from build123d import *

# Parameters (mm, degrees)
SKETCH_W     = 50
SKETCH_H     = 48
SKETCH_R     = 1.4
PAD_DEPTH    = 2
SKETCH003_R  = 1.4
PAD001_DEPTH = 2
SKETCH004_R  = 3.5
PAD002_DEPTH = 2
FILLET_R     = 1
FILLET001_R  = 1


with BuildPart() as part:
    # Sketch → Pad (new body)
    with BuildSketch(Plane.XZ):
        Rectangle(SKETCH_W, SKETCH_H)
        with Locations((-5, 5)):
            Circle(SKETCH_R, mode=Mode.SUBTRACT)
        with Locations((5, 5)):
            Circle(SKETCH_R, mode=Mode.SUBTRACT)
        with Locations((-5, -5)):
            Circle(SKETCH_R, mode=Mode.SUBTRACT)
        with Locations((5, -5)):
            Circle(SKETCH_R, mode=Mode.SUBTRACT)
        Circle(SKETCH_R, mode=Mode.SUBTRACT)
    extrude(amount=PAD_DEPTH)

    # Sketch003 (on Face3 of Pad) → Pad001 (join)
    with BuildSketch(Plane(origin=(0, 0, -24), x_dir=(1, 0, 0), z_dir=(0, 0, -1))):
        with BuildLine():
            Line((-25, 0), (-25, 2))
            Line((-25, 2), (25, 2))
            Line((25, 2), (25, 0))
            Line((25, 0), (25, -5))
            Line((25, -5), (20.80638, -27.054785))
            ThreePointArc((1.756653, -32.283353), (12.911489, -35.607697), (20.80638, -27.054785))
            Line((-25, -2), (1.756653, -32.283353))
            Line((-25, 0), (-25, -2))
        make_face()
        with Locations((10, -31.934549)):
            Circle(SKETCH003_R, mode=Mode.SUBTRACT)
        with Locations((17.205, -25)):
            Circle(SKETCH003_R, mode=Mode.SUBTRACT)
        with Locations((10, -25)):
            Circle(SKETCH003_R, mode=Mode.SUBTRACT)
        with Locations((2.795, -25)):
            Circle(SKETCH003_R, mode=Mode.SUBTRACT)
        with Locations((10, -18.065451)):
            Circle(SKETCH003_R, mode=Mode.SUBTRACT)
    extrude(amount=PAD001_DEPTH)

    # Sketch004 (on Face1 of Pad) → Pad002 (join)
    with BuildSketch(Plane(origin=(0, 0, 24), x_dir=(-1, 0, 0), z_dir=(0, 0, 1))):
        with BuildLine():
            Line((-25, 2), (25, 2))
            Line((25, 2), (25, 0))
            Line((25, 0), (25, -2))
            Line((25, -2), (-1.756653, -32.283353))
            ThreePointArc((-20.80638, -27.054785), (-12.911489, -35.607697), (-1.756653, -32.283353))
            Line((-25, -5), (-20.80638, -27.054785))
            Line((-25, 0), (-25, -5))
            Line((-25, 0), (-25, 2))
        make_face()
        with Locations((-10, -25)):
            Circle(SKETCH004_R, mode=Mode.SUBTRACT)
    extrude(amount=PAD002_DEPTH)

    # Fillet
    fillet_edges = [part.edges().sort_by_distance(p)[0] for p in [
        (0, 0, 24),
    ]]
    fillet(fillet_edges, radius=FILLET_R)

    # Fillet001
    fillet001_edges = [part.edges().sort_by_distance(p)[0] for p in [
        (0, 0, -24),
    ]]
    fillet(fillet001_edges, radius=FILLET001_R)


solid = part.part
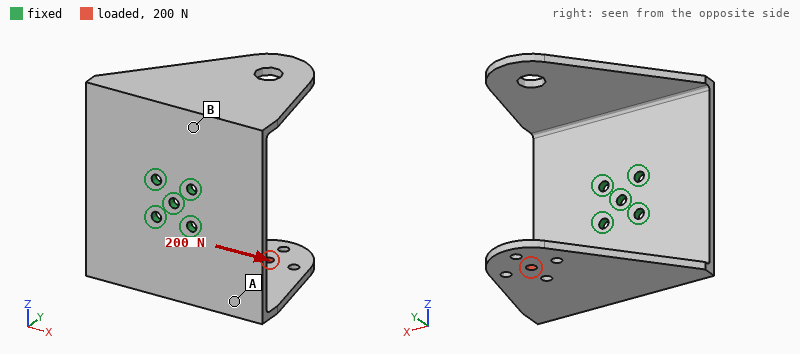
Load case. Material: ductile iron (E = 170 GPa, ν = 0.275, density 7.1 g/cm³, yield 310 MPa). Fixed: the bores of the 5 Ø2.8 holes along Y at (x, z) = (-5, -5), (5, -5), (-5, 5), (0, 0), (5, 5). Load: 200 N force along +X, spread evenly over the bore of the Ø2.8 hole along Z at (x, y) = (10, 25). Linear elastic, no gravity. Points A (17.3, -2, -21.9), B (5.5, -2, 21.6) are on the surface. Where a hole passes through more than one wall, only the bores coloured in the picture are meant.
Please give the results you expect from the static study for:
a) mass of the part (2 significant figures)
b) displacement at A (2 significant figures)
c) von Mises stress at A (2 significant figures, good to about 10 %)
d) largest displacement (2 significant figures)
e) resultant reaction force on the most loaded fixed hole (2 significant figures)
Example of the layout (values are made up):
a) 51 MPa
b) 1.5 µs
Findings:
a) 69 g
b) 0.12 mm
c) 53 MPa
d) 0.31 mm
e) 380 N
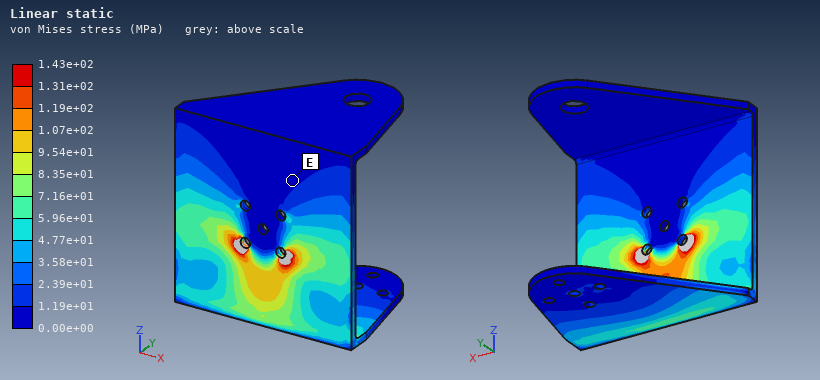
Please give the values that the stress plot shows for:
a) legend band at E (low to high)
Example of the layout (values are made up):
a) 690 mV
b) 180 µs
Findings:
a) 0.00e+00 to 1.19e+01 MPa
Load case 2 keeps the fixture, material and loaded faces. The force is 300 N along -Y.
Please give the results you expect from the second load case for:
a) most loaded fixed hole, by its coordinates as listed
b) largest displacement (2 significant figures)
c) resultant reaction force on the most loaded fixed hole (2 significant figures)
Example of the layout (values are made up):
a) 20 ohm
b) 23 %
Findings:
a) (5, -5)
b) 0.53 mm
c) 470 N
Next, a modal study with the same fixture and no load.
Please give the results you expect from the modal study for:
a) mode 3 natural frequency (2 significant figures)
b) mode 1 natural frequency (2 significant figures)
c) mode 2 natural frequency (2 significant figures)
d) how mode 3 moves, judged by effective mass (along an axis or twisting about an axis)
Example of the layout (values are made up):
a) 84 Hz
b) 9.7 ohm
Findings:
a) 1400 Hz
b) 870 Hz
c) 880 Hz
d) along X
